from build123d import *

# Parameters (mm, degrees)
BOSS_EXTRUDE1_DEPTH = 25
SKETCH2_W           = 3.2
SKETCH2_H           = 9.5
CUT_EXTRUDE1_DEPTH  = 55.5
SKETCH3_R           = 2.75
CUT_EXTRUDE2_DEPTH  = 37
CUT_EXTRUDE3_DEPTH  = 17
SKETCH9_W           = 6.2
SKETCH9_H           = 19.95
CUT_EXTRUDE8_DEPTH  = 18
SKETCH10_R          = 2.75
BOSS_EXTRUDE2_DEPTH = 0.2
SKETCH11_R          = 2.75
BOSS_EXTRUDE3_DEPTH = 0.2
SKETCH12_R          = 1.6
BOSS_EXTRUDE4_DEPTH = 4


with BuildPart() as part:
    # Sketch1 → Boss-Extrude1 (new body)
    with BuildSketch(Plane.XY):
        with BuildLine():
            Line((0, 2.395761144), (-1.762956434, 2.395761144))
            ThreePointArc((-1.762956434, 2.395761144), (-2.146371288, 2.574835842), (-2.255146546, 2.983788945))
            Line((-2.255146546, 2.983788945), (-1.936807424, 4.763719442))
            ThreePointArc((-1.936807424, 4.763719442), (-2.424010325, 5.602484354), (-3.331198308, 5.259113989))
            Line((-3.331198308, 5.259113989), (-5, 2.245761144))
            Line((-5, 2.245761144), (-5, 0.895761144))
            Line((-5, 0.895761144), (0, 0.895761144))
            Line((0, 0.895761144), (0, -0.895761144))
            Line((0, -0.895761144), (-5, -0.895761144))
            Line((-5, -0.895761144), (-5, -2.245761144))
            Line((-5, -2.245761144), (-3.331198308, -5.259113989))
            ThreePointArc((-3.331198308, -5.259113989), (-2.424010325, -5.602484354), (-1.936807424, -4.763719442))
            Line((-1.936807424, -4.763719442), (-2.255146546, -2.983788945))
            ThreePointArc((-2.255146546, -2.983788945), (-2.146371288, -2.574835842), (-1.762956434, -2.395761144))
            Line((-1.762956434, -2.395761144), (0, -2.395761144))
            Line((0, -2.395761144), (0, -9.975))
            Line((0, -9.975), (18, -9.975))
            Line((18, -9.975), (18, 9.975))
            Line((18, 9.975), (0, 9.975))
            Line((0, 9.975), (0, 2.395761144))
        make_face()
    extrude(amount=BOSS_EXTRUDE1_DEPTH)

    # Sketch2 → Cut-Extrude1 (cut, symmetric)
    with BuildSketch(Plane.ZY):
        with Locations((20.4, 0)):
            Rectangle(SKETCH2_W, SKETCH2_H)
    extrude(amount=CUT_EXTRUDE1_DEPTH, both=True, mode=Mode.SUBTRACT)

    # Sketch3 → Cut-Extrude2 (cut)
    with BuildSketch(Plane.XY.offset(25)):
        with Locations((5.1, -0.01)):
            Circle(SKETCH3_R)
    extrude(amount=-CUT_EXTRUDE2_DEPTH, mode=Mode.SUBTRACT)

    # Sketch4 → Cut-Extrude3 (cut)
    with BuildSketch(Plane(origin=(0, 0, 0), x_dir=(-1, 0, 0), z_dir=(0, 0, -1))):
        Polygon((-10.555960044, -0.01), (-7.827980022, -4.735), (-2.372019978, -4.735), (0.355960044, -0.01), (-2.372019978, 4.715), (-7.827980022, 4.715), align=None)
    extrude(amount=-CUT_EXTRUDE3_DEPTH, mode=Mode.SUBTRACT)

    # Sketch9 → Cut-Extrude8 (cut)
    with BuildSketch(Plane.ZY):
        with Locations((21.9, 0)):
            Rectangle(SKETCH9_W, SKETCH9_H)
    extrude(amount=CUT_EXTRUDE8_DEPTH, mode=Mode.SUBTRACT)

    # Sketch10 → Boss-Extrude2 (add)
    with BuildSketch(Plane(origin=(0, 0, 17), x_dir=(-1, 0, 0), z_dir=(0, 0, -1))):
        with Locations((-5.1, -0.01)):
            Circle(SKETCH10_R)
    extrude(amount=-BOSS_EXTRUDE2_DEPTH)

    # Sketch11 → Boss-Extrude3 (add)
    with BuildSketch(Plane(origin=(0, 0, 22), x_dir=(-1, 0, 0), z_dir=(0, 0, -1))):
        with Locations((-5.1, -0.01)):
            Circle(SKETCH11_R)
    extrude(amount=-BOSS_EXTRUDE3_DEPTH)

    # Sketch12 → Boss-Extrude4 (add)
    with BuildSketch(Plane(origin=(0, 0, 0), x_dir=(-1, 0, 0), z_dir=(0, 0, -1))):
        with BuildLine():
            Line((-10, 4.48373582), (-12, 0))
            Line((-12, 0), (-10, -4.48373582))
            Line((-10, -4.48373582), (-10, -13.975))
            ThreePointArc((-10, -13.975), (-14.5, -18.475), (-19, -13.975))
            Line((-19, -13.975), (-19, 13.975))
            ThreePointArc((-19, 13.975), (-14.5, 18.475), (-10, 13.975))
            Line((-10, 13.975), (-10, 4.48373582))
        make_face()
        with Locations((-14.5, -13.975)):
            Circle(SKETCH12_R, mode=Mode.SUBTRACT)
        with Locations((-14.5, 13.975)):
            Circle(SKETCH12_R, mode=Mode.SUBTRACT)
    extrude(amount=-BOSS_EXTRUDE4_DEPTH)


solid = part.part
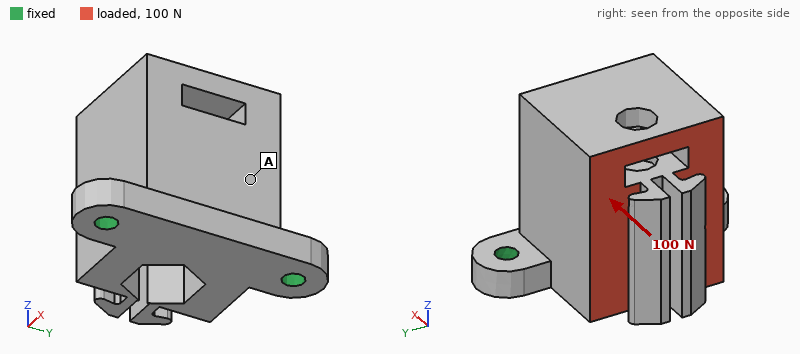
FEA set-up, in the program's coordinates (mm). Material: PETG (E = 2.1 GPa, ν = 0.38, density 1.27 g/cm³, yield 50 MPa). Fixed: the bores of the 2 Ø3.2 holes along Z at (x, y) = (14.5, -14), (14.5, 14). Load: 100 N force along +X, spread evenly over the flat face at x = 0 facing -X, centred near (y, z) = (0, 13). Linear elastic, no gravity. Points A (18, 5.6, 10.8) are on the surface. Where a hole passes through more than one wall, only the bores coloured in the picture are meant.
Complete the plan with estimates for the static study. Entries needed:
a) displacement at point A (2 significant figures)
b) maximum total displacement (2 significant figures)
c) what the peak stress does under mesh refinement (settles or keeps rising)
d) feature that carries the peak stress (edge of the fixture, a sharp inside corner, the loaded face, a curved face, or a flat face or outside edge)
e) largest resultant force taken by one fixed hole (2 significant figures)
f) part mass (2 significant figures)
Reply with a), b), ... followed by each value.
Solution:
a) 0.20 mm
b) 0.56 mm
c) keeps rising
d) edge of the fixture
e) 51 N
f) 10 g
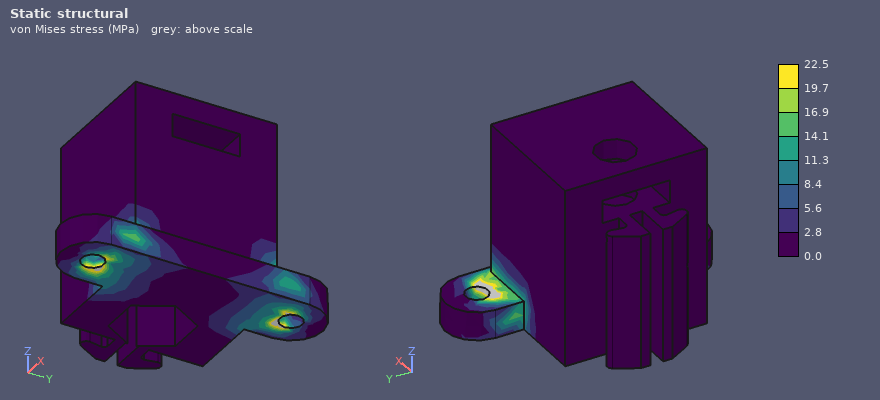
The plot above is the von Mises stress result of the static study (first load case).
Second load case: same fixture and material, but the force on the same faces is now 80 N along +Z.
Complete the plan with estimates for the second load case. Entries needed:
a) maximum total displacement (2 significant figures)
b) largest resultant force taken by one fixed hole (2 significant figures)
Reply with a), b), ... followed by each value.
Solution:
a) 0.60 mm
b) 44 N
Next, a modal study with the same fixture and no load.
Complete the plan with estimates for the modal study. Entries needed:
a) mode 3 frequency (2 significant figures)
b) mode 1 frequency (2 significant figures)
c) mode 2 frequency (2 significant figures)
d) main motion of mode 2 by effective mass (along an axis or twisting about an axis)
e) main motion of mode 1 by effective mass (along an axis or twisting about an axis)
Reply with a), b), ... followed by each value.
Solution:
a) 3100 Hz
b) 780 Hz
c) 2500 Hz
d) along Y
e) along X
